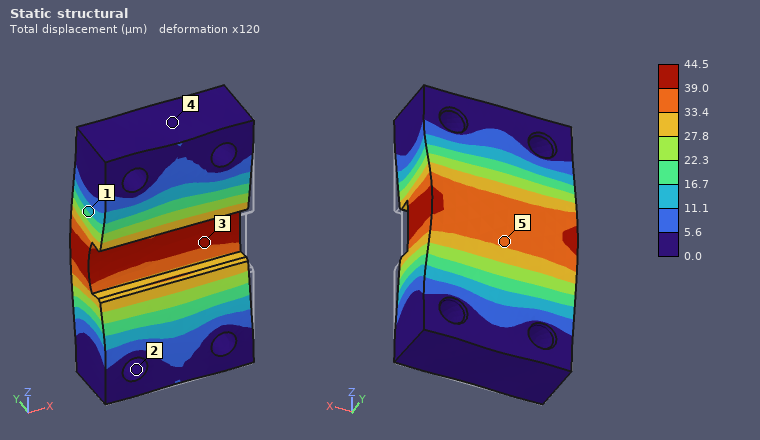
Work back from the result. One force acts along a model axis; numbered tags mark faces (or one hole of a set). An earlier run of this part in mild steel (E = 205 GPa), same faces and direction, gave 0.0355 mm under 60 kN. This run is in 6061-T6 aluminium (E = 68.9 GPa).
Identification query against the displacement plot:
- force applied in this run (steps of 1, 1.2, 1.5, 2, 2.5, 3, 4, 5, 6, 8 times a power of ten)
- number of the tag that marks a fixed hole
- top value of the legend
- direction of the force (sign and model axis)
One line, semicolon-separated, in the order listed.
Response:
25 kN; 2; 44.5 µm; +Y
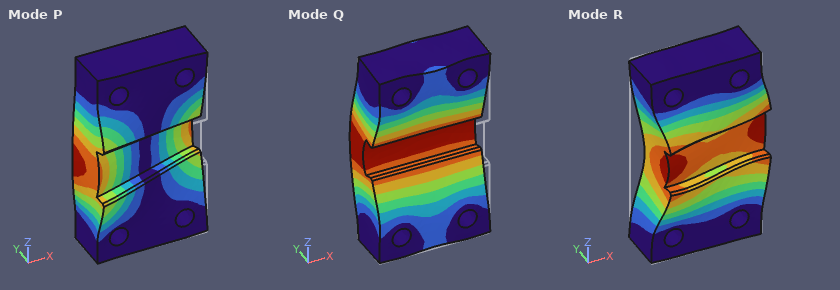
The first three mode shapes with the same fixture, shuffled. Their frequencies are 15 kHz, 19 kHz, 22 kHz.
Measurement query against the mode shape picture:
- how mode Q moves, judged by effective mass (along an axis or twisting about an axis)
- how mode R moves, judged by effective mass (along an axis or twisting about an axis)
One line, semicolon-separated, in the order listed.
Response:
along Y; along X
